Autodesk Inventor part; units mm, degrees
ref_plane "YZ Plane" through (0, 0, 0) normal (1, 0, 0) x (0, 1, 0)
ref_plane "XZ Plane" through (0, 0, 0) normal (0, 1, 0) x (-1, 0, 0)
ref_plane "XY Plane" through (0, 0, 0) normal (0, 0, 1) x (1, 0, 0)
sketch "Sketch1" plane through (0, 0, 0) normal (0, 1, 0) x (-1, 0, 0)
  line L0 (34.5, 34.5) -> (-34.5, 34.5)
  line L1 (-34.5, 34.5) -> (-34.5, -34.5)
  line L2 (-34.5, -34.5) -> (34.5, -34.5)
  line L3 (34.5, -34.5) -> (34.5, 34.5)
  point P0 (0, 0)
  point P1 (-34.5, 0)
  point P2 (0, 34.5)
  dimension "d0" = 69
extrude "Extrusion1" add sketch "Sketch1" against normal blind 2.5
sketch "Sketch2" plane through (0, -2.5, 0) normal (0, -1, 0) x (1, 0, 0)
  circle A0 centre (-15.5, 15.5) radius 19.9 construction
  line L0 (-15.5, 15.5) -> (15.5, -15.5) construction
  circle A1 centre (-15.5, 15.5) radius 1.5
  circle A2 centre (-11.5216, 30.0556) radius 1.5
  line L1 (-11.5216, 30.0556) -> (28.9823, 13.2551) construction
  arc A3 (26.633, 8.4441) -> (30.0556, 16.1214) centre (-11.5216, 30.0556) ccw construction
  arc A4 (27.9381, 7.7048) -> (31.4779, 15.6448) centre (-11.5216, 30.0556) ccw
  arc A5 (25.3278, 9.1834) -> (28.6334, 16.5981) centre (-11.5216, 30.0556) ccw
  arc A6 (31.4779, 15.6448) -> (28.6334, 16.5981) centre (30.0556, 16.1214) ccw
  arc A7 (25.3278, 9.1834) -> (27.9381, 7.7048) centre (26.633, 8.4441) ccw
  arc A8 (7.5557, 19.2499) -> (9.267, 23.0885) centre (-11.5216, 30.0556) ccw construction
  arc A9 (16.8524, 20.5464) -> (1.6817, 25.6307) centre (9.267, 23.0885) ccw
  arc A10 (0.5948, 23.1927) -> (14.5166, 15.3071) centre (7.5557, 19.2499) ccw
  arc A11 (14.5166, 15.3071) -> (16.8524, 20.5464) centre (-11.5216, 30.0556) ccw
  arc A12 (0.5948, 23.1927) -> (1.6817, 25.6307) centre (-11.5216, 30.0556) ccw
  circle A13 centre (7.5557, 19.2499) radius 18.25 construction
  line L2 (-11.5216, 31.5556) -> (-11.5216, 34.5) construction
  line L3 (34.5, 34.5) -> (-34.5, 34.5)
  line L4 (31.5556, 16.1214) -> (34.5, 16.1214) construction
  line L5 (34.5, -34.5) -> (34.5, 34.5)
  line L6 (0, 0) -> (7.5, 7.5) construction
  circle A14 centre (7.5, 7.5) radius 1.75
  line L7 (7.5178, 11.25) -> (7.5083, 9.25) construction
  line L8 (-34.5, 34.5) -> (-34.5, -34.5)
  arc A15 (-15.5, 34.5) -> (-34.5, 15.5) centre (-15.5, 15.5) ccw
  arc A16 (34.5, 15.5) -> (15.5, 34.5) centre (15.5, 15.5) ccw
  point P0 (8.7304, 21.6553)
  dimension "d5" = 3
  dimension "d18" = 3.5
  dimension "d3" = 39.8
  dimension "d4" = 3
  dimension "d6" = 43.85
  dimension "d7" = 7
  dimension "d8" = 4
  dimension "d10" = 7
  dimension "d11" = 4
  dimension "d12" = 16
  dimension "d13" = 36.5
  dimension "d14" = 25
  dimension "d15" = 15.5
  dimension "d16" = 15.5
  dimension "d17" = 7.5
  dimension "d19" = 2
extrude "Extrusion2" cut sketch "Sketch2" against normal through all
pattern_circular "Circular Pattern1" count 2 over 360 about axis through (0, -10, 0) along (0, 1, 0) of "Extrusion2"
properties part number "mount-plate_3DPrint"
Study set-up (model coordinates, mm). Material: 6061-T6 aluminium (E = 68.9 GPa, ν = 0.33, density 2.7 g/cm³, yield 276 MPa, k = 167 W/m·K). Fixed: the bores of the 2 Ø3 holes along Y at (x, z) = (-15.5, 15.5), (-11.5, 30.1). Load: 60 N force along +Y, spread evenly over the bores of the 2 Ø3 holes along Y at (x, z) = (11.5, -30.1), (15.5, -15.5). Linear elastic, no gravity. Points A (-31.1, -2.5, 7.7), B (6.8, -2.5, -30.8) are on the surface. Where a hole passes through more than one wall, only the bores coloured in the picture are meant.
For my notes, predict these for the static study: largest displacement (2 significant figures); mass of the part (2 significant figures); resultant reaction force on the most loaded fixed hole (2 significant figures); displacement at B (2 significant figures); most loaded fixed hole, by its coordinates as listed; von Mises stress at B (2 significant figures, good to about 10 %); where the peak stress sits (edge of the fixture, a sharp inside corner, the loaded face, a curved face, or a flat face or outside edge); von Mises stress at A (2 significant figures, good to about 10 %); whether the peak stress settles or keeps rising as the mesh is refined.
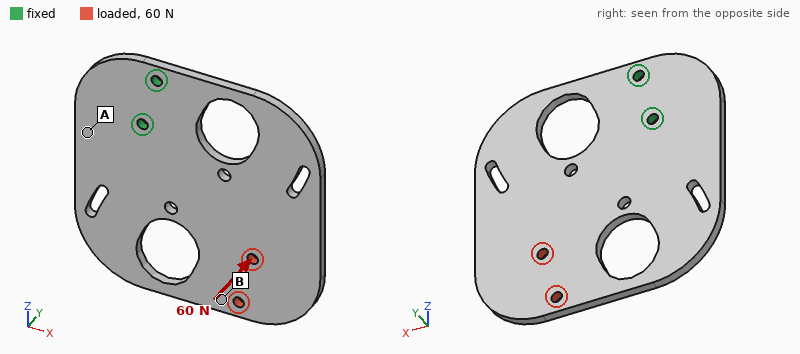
0.96 mm
26 g
120 N
0.70 mm
(-15.5, 15.5)
11 MPa
edge of the fixture
28 MPa
keeps rising
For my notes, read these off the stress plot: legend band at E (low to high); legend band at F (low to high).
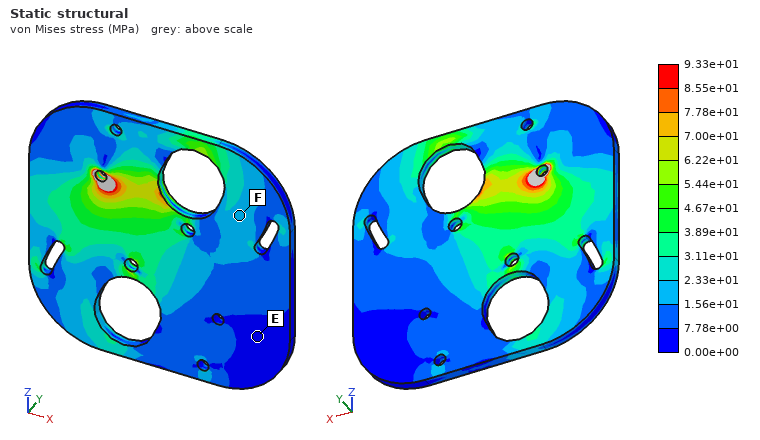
0.00e+00 to 7.78e+00 MPa
1.56e+01 to 2.33e+01 MPa
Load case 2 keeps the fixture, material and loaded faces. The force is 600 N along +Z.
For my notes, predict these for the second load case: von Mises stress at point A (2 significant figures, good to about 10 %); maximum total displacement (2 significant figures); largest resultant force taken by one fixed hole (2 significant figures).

12 MPa
74 µm
1.0 kN
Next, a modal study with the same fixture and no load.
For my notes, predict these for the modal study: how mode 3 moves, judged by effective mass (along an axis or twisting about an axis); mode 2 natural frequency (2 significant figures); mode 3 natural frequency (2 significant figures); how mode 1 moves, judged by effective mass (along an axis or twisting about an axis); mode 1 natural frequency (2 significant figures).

along Y
960 Hz
1800 Hz
along Y
510 Hz
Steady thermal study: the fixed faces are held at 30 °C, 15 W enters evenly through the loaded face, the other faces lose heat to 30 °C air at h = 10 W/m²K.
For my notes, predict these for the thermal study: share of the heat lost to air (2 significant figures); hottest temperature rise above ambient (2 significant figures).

13 %
53 K
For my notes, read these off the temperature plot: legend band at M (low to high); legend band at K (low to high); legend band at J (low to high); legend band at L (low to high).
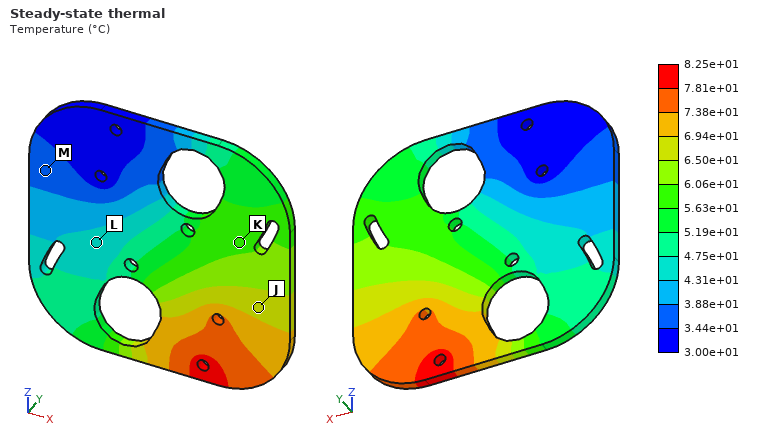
3.44e+01 to 3.88e+01 °C
5.63e+01 to 6.06e+01 °C
6.50e+01 to 6.94e+01 °C
4.31e+01 to 4.75e+01 °C
